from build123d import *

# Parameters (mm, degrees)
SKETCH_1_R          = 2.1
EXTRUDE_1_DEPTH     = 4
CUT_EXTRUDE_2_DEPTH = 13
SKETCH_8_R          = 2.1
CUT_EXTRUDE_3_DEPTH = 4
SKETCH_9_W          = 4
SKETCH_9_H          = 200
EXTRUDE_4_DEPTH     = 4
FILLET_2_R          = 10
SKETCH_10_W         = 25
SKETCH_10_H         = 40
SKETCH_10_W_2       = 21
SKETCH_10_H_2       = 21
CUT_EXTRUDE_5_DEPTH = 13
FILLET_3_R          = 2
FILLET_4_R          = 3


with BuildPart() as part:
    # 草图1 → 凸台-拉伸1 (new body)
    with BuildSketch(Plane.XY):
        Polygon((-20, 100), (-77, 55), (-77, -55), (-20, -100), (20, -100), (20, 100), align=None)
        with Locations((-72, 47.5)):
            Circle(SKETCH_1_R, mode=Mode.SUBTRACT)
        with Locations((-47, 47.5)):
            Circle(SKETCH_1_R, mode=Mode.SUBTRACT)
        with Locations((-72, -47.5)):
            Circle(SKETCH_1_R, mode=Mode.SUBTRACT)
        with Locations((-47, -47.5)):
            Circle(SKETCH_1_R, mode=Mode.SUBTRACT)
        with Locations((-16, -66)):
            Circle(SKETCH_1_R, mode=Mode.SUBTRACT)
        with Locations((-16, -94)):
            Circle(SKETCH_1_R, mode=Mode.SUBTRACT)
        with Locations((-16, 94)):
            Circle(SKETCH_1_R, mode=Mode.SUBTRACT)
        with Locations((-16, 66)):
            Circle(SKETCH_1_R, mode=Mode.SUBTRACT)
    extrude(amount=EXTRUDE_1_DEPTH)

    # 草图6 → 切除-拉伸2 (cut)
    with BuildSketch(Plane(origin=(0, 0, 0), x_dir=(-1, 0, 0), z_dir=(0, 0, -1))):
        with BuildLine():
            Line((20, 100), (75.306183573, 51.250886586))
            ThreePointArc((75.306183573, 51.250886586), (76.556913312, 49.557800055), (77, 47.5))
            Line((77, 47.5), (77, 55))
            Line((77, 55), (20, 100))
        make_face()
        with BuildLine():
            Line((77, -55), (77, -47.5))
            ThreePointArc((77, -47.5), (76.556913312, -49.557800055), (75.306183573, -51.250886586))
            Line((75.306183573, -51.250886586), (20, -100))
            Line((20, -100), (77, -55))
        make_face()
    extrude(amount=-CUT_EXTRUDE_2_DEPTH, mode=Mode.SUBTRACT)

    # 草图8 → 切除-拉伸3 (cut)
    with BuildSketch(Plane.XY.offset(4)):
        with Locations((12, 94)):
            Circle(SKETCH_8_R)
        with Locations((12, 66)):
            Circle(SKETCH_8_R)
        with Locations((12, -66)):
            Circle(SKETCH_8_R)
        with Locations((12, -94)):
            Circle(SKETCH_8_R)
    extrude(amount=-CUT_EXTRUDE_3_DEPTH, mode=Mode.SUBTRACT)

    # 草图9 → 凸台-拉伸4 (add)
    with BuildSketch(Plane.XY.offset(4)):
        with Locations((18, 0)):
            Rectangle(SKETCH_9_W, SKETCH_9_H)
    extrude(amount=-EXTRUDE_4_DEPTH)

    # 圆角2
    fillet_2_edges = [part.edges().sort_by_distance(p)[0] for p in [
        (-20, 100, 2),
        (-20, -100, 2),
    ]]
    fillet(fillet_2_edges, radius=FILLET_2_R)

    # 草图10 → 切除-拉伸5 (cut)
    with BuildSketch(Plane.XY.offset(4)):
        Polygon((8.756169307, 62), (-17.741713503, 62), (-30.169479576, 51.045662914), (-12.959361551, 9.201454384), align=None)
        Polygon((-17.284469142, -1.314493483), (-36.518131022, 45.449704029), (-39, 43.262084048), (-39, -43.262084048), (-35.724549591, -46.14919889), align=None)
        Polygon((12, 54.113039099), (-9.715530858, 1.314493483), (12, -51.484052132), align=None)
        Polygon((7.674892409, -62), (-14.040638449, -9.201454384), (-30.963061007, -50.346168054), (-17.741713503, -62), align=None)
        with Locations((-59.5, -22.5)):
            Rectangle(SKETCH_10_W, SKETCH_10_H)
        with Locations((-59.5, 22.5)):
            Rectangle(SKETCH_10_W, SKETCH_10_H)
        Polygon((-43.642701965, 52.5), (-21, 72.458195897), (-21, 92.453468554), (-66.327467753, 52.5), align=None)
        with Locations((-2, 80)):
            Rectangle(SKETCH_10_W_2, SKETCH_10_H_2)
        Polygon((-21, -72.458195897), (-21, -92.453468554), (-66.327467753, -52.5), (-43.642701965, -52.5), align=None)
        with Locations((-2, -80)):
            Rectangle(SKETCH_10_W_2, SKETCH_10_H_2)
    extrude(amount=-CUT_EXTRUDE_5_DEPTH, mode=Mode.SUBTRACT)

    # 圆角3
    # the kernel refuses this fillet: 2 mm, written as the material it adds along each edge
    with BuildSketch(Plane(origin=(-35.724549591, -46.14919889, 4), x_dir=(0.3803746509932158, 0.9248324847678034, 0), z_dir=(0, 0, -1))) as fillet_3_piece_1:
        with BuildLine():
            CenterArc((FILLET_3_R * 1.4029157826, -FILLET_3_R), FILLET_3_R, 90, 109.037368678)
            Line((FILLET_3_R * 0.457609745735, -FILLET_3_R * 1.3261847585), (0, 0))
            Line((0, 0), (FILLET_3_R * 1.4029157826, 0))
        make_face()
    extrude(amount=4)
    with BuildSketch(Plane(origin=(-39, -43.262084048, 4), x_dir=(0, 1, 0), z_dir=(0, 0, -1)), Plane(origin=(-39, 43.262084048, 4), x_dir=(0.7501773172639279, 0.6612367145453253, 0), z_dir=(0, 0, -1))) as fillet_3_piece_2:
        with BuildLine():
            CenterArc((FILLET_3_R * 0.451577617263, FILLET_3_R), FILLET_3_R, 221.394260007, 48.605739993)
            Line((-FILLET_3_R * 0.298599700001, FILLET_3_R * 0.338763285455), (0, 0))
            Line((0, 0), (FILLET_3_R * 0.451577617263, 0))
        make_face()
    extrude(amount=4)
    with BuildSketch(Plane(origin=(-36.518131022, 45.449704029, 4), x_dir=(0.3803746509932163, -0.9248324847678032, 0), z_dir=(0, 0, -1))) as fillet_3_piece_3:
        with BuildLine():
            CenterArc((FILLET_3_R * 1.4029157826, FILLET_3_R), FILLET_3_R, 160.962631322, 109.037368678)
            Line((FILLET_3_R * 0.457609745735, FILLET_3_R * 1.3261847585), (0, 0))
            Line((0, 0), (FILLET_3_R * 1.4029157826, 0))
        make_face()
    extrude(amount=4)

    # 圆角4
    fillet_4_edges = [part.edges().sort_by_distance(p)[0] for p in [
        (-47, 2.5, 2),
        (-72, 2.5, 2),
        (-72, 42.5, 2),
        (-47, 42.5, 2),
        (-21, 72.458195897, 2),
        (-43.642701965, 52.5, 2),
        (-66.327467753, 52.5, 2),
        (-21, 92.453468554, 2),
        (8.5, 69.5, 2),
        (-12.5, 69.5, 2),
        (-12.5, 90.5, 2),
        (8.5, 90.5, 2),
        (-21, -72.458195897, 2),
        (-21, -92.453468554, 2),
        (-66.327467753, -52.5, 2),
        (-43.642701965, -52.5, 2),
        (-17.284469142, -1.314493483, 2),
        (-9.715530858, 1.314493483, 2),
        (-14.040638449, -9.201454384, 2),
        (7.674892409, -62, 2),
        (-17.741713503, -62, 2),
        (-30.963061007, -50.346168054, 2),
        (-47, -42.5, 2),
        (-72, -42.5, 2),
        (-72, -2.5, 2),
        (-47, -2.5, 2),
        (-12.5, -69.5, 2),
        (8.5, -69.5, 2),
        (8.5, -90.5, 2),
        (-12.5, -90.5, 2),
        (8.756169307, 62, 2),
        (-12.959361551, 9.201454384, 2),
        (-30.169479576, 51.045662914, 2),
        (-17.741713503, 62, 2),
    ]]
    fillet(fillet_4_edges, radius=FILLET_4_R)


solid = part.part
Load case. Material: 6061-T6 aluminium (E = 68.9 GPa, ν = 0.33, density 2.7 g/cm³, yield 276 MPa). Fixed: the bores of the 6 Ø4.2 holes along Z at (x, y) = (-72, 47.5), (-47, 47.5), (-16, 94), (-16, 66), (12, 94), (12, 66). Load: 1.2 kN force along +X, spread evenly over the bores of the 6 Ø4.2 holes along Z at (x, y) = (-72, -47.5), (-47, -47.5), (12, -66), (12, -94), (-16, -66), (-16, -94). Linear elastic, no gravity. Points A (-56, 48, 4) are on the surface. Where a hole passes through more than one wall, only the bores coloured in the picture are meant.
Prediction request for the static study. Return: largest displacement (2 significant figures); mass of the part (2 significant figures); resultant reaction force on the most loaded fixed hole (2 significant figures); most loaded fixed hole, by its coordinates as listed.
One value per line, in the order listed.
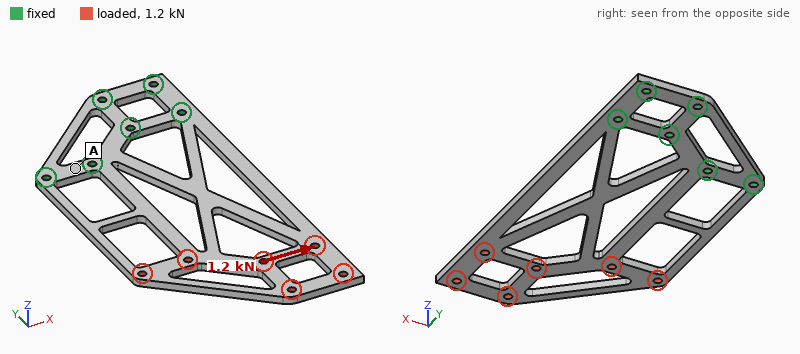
0.41 mm
85 g
2.2 kN
(12, 66)
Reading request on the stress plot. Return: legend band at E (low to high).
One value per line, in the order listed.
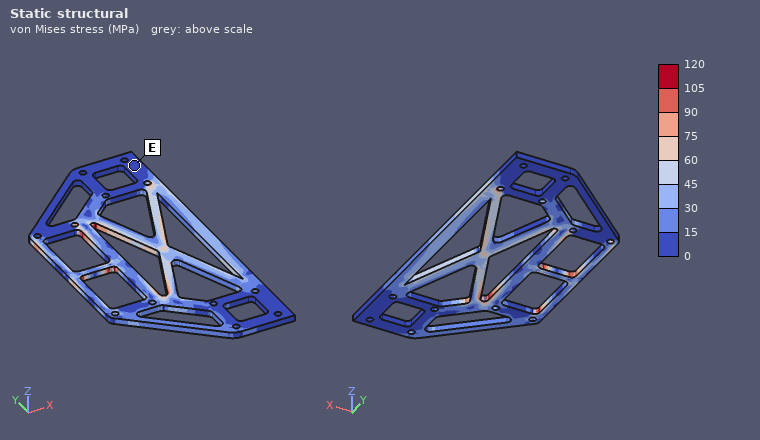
0 to 15 MPa
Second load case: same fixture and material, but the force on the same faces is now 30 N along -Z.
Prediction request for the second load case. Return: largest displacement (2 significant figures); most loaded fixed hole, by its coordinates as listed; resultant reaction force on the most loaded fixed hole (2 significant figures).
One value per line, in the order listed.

2.2 mm
(-47, 47.5)
41 N
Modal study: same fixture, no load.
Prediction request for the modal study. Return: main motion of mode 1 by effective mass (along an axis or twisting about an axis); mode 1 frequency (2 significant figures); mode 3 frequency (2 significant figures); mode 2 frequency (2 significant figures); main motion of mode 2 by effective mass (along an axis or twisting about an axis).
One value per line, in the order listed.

along Z
130 Hz
770 Hz
440 Hz
twisting about Y
